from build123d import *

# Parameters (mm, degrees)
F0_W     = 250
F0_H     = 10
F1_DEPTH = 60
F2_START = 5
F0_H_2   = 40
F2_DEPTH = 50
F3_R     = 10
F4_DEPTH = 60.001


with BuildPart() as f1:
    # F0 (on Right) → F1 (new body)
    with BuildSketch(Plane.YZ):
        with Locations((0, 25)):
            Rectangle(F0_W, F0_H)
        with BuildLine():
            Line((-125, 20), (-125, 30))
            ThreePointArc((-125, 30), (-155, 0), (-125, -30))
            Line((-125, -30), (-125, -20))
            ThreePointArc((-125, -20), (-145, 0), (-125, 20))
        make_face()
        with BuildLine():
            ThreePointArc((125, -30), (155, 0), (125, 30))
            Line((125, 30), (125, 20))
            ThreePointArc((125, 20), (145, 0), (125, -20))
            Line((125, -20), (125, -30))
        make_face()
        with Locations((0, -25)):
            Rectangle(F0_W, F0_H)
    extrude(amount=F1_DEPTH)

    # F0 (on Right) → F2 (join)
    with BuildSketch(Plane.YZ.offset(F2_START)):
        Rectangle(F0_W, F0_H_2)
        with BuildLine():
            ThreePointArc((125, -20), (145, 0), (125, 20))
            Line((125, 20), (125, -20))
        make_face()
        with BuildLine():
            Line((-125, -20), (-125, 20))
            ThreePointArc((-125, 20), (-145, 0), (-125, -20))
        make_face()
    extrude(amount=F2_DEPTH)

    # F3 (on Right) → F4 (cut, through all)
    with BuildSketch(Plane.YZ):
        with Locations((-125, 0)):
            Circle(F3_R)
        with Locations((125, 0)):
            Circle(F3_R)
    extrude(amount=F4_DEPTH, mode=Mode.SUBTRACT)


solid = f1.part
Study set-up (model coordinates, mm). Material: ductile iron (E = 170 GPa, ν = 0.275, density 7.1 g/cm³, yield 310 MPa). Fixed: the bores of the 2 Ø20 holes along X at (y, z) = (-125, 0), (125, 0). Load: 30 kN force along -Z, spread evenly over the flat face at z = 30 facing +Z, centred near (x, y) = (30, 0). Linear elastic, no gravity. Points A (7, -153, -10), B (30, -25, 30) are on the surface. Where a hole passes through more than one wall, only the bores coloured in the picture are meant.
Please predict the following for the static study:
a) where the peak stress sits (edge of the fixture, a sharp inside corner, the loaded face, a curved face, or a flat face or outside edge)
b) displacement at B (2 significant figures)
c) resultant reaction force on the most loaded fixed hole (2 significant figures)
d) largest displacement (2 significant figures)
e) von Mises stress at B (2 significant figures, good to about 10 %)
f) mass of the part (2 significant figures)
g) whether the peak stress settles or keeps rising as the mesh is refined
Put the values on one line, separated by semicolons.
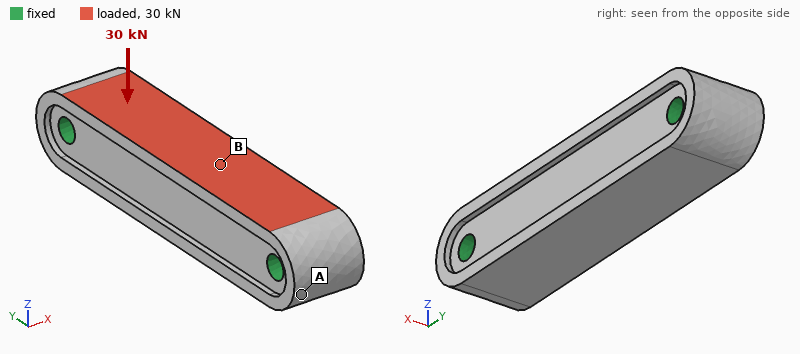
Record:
edge of the fixture; 16 µm; 15 kN; 17 µm; 12 MPa; 6.6 kg; keeps rising
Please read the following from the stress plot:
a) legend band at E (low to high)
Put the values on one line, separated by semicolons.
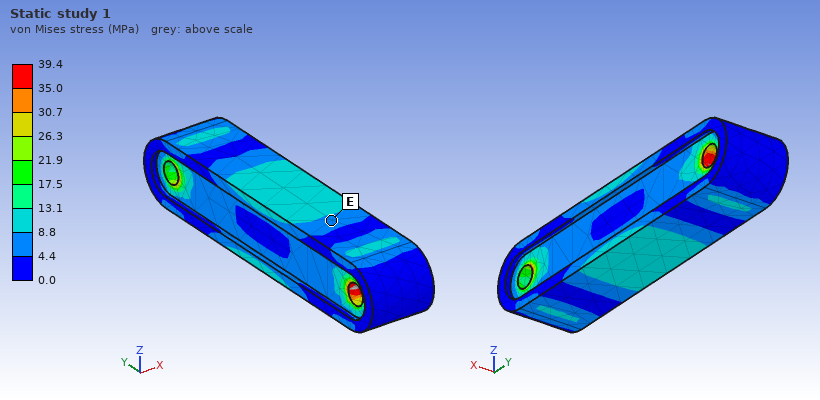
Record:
4.4 to 8.8 MPa
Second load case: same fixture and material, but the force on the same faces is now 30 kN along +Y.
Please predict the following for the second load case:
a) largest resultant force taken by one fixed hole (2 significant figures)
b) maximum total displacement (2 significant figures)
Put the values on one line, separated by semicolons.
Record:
15 kN; 2.6 µm
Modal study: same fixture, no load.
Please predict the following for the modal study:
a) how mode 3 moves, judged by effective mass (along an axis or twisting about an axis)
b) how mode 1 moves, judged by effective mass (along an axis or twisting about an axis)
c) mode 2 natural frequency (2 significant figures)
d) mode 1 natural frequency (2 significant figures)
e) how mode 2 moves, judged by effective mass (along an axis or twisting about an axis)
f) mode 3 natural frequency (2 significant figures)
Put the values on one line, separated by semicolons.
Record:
twisting about Y; along Z; 3400 Hz; 3100 Hz; along X; 5200 Hz
